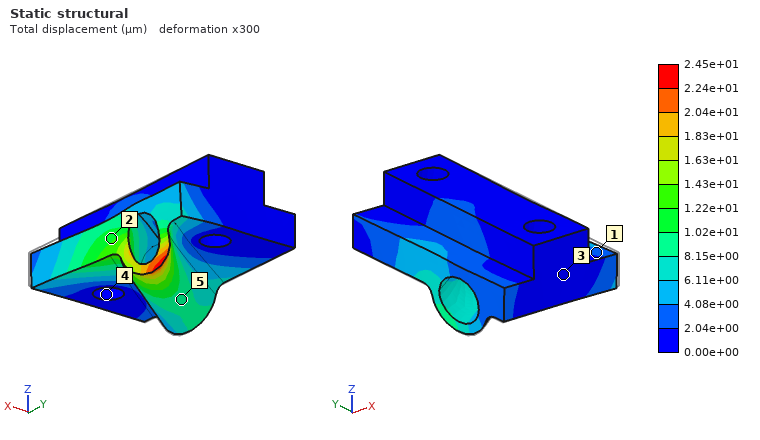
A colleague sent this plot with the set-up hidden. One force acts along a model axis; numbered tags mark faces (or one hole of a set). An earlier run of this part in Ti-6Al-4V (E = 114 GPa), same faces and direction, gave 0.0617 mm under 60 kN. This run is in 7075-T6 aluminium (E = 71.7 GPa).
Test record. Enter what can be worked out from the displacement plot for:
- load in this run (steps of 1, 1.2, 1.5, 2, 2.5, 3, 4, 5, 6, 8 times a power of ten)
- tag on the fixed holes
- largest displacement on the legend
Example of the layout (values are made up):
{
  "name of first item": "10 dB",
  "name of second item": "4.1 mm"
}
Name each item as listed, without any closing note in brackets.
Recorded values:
{
  "load in this run": "15 kN",
  "tag on the fixed holes": "4",
  "largest displacement on the legend": "2.45e+01 µm"
}
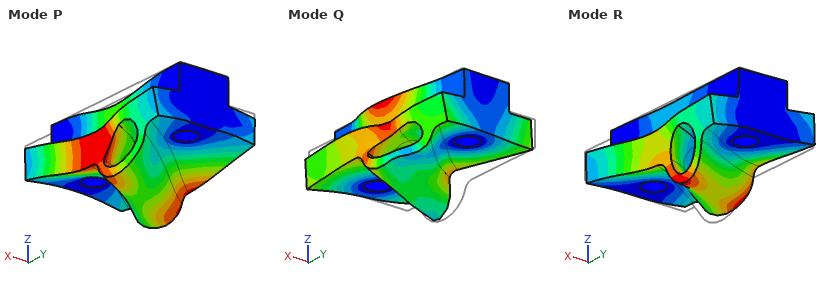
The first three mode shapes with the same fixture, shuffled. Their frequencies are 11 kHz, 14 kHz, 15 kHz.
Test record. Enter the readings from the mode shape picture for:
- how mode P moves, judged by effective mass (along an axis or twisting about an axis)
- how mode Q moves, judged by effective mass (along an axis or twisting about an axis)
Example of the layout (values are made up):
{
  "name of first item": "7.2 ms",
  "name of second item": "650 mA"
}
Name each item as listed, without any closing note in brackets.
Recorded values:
{
  "how mode P moves, judged by effective mass": "along Z",
  "how mode Q moves, judged by effective mass": "along X"
}
